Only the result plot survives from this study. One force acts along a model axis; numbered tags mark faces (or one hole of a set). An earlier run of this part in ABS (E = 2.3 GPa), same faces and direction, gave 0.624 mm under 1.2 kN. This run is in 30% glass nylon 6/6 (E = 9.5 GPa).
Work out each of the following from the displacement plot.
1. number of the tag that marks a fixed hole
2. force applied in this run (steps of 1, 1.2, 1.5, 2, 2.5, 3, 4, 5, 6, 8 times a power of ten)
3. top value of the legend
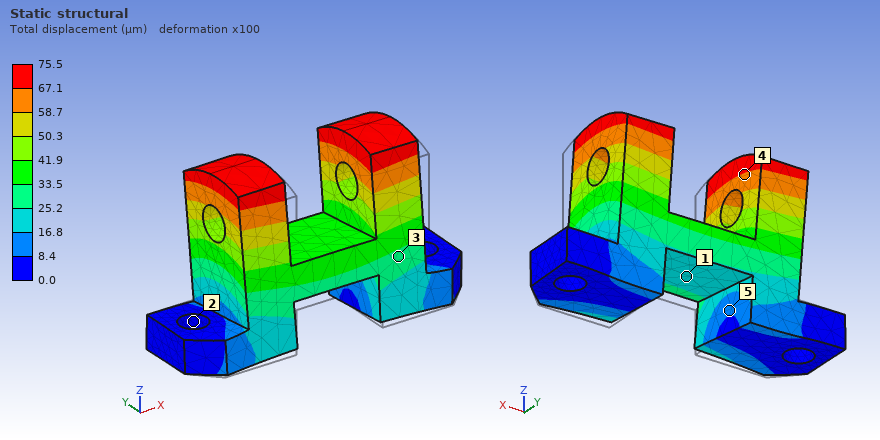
2
600 N
75.5 µm
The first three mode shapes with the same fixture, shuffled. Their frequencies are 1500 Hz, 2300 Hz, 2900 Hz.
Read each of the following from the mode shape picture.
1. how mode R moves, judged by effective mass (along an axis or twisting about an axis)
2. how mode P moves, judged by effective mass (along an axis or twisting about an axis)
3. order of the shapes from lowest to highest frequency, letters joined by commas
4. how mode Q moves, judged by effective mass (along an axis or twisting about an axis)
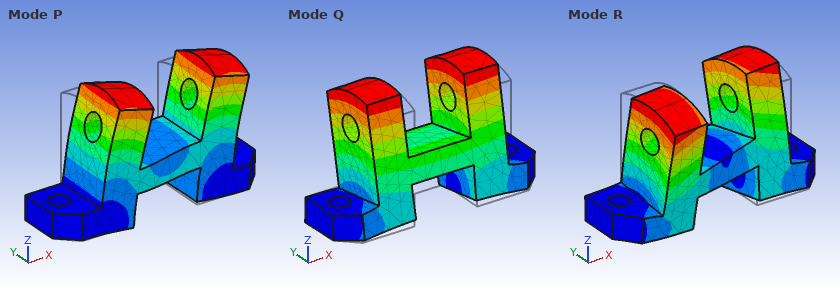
twisting about Z
along X
Q, R, P
along Y
